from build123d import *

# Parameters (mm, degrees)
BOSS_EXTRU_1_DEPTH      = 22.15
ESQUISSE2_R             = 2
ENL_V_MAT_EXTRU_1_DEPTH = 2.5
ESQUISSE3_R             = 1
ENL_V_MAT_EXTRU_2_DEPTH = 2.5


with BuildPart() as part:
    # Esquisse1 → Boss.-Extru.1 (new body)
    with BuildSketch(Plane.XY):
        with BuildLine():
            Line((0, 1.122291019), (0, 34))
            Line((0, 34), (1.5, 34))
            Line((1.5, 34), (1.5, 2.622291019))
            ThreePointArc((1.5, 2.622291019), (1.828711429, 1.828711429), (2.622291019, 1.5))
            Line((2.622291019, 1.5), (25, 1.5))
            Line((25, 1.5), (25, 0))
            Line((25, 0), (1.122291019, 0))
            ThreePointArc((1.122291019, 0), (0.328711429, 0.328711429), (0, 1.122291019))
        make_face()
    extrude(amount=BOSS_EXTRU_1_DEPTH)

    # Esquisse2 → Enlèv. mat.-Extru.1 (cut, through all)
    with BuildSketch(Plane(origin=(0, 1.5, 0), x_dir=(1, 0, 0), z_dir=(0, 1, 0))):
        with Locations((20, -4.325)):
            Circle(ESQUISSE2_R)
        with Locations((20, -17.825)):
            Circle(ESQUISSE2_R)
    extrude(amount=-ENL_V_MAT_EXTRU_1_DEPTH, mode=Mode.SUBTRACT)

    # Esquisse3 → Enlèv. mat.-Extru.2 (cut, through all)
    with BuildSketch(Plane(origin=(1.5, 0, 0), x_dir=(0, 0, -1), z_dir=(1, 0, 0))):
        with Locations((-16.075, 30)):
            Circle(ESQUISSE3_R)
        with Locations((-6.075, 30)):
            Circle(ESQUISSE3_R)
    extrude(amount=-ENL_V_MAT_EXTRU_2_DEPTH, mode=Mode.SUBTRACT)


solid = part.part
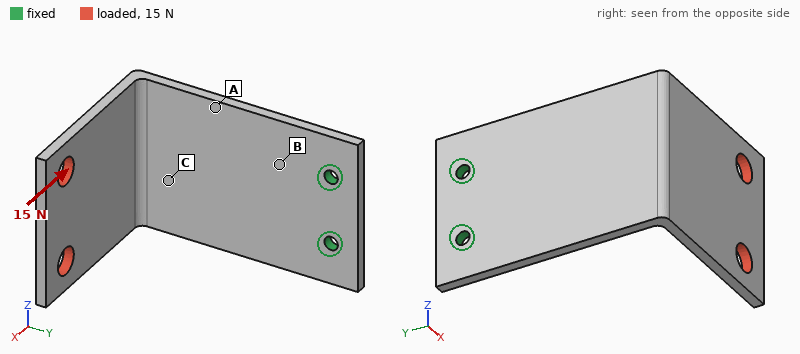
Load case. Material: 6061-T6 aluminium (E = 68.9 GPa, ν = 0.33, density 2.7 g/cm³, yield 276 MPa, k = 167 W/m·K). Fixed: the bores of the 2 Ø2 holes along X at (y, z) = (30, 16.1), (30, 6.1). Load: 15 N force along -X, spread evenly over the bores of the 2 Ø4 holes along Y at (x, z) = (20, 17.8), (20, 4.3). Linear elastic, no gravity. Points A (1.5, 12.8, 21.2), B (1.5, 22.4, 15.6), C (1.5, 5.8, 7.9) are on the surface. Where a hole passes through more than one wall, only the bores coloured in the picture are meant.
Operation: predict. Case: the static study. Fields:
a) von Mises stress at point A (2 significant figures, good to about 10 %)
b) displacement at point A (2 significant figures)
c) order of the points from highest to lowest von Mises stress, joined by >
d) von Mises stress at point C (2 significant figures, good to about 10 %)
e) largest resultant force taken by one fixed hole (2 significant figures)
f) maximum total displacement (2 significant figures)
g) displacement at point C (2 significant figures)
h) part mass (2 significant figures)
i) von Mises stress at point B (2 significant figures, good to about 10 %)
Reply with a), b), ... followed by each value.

a) 23 MPa
b) 0.11 mm
c) B > A > C
d) 8.9 MPa
e) 7.5 N
f) 0.45 mm
g) 0.21 mm
h) 5.0 g
i) 35 MPa
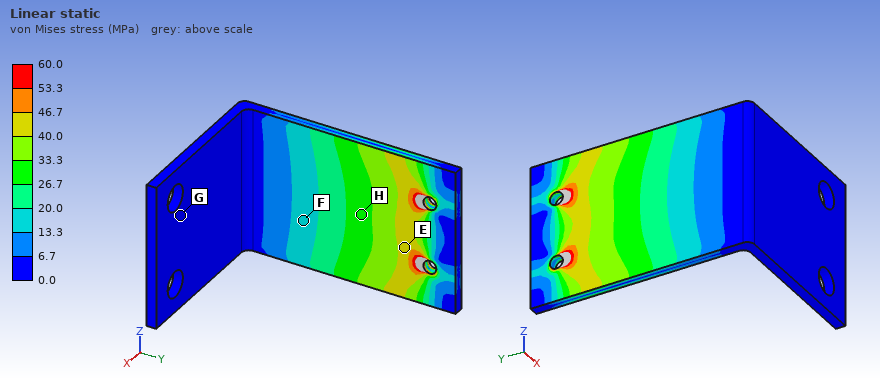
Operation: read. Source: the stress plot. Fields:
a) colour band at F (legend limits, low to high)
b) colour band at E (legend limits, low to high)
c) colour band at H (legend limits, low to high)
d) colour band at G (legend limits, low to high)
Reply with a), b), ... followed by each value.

a) 13.3 to 20.0 MPa
b) 40.0 to 46.7 MPa
c) 26.7 to 33.3 MPa
d) 0.0 to 6.7 MPa
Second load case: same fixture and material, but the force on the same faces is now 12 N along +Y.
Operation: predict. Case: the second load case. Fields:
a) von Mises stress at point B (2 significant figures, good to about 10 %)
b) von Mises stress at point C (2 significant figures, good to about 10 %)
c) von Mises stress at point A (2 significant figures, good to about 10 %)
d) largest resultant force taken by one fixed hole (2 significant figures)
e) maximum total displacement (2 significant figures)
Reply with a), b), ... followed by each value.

a) 26 MPa
b) 26 MPa
c) 29 MPa
d) 6.0 N
e) 0.49 mm
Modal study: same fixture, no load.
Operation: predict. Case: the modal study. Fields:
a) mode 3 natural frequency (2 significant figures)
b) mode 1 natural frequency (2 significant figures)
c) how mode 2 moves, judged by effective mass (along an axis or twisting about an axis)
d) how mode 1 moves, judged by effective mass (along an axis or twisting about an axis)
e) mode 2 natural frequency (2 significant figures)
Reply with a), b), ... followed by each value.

a) 1800 Hz
b) 590 Hz
c) along Z
d) along X
e) 1200 Hz
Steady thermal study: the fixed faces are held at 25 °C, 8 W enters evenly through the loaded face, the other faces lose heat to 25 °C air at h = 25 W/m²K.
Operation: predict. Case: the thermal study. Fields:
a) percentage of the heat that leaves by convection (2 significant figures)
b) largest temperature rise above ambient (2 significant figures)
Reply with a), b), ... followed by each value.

a) 24 %
b) 61 K
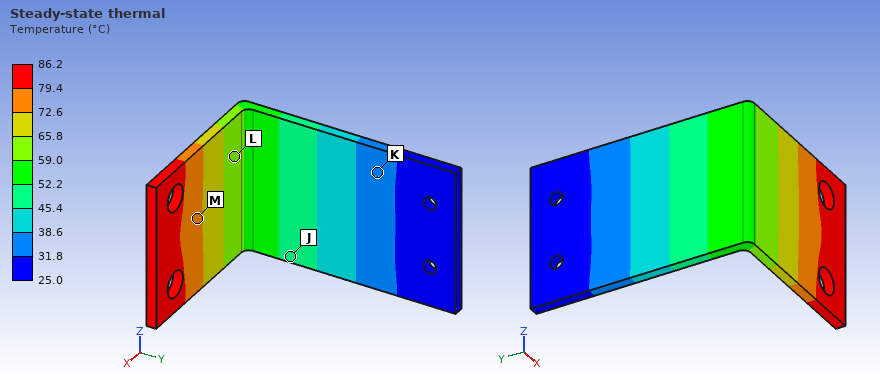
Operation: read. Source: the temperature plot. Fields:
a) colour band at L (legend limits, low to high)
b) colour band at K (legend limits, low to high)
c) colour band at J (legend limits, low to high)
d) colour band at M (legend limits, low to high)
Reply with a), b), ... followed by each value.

a) 59.0 to 65.8 °C
b) 31.8 to 38.6 °C
c) 45.4 to 52.2 °C
d) 72.6 to 79.4 °C
